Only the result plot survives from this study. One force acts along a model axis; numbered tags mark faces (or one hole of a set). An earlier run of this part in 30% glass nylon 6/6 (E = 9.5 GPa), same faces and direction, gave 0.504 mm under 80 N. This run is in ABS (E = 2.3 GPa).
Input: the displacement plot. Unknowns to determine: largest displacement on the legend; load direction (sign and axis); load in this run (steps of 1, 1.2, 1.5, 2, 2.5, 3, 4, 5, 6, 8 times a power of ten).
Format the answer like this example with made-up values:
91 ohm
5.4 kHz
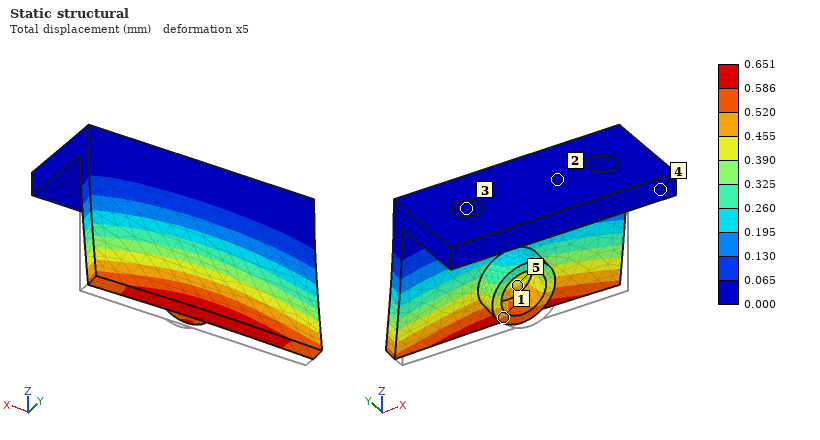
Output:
0.651 mm
+Y
25 N
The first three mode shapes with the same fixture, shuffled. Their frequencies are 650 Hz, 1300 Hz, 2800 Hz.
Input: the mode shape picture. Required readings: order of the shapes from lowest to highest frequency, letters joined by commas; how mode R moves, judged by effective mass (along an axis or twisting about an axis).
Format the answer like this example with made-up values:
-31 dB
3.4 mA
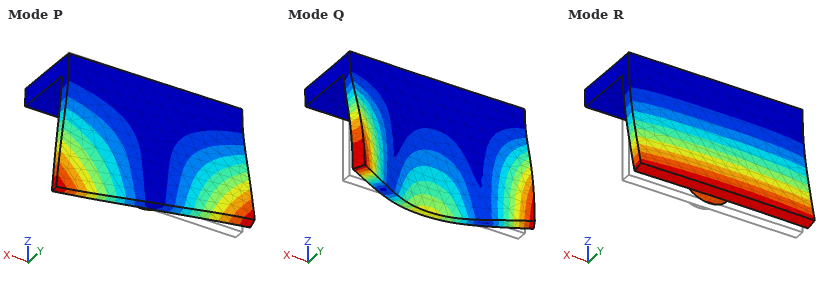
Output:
R, P, Q
along Y
